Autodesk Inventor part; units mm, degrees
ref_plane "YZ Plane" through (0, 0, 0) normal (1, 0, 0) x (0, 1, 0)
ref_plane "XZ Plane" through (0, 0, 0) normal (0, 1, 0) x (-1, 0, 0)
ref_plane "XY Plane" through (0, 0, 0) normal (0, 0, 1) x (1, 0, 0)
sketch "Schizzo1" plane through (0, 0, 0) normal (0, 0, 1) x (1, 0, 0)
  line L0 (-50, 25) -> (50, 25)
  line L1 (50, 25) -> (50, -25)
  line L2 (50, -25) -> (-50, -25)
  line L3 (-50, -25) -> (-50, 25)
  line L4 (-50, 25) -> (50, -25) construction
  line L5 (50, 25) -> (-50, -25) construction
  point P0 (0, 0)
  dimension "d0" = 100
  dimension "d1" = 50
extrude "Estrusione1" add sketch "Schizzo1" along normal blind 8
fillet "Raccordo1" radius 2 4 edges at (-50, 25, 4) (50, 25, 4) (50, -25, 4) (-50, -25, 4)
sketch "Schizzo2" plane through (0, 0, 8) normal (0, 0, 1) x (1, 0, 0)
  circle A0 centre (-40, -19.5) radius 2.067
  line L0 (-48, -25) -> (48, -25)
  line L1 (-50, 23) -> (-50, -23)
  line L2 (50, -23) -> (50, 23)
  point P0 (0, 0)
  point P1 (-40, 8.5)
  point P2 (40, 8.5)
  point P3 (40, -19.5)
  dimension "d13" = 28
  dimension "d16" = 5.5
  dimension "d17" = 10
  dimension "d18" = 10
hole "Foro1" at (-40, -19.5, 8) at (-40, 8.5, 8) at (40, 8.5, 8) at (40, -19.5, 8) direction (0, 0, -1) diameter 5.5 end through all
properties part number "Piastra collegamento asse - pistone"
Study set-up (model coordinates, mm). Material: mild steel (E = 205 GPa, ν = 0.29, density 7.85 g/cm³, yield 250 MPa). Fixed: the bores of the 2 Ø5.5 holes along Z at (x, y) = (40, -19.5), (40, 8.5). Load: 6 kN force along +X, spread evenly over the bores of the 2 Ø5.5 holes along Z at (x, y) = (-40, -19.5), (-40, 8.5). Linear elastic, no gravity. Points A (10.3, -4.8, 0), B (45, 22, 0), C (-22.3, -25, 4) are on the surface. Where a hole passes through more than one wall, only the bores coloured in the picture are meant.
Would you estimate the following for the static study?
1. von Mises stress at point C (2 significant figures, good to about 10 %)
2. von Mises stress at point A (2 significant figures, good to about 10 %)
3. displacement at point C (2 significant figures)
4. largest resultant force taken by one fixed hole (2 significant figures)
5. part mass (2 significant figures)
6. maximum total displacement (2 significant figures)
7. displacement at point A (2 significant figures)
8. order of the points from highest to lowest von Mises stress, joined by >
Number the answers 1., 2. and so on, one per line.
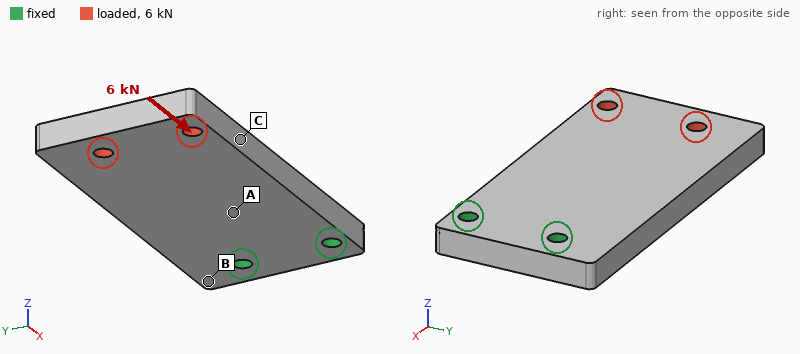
1. 27 MPa
2. 17 MPa
3. 8.4 µm
4. 3.1 kN
5. 310 g
6. 13 µm
7. 2.8 µm
8. C > A > B
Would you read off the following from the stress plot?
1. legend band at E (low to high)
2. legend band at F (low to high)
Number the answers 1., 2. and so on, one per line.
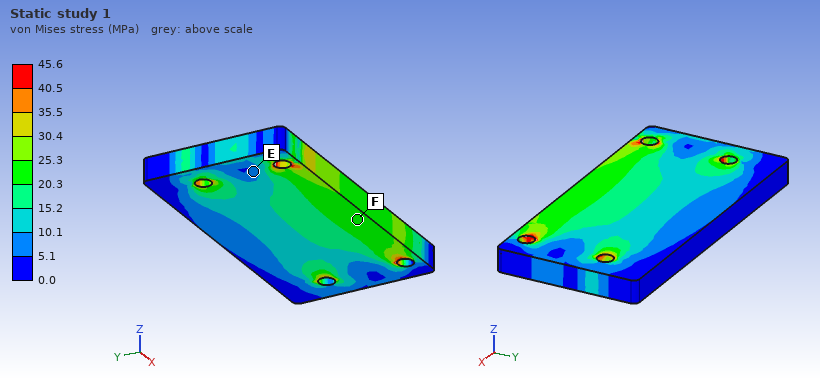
1. 5.1 to 10.1 MPa
2. 20.3 to 25.3 MPa
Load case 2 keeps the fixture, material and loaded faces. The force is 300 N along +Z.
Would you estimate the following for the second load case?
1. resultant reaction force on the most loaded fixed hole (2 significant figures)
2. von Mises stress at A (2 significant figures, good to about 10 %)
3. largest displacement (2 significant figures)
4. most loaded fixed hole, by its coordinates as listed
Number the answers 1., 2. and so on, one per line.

1. 180 N
2. 27 MPa
3. 0.15 mm
4. (40, 8.5)
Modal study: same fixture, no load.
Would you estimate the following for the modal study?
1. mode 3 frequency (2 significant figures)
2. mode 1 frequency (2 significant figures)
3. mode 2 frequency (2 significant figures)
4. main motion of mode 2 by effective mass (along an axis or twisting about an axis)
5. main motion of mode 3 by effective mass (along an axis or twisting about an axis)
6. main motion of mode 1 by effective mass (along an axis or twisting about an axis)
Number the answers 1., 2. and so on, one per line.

1. 3800 Hz
2. 810 Hz
3. 3000 Hz
4. twisting about X
5. along Y
6. along Z
